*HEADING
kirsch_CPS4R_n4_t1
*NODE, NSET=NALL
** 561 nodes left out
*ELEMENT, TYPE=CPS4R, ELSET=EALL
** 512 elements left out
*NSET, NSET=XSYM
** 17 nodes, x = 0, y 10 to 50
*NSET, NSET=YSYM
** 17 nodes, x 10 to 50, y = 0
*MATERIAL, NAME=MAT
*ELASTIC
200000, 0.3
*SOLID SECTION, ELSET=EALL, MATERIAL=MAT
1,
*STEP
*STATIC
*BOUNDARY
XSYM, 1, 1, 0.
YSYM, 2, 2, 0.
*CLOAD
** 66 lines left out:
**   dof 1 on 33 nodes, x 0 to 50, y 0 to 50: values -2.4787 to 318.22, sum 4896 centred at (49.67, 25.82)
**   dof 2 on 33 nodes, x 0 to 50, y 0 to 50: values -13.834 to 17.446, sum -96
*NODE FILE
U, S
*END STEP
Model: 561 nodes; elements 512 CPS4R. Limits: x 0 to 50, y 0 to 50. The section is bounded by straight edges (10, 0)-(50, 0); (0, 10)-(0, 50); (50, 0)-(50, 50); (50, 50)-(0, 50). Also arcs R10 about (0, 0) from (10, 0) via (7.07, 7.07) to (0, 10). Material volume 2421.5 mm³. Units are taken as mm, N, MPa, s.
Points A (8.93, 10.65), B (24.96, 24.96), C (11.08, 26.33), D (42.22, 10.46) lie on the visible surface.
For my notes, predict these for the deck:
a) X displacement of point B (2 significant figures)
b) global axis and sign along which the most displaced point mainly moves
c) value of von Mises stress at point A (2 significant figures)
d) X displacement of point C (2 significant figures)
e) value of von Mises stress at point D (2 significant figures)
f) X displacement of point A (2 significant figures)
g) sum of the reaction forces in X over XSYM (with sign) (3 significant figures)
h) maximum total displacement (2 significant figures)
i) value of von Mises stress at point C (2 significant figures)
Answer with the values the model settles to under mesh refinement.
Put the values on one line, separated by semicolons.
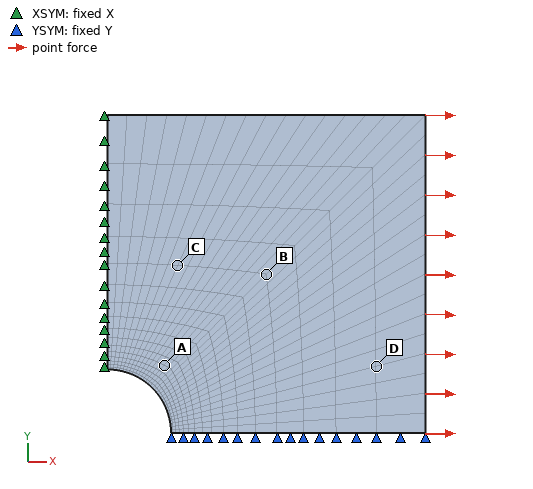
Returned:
0.014 mm; +X; 130 MPa; 0.0060 mm; 90 MPa; 0.0081 mm; -4900 N; 0.028 mm; 110 MPa
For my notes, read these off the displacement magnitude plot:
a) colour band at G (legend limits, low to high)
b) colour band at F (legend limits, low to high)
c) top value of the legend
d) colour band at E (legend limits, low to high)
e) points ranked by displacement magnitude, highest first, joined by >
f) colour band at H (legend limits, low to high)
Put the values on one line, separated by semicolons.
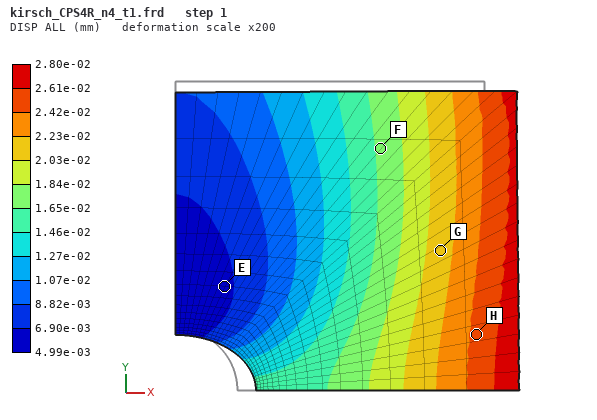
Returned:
2.03e-02 to 2.23e-02 mm; 1.65e-02 to 1.84e-02 mm; 2.80e-02 mm; 4.99e-03 to 6.90e-03 mm; H > G > F > E; 2.42e-02 to 2.61e-02 mm
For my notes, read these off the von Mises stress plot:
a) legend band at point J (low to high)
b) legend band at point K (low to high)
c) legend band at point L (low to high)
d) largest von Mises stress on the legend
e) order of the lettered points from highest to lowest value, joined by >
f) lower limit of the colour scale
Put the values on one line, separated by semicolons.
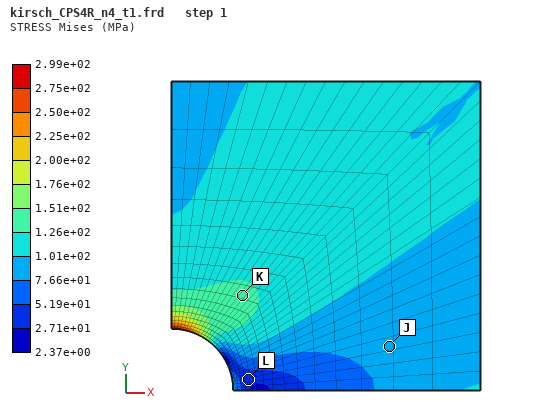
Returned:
7.66e+01 to 1.01e+02 MPa; 1.26e+02 to 1.51e+02 MPa; 2.71e+01 to 5.19e+01 MPa; 2.99e+02 MPa; K > J > L; 2.37e+00 MPa
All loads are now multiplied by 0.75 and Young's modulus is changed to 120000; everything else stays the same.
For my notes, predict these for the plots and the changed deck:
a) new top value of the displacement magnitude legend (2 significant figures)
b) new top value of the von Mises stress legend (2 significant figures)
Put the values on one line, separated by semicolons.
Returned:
0.035 mm; 220 MPa
